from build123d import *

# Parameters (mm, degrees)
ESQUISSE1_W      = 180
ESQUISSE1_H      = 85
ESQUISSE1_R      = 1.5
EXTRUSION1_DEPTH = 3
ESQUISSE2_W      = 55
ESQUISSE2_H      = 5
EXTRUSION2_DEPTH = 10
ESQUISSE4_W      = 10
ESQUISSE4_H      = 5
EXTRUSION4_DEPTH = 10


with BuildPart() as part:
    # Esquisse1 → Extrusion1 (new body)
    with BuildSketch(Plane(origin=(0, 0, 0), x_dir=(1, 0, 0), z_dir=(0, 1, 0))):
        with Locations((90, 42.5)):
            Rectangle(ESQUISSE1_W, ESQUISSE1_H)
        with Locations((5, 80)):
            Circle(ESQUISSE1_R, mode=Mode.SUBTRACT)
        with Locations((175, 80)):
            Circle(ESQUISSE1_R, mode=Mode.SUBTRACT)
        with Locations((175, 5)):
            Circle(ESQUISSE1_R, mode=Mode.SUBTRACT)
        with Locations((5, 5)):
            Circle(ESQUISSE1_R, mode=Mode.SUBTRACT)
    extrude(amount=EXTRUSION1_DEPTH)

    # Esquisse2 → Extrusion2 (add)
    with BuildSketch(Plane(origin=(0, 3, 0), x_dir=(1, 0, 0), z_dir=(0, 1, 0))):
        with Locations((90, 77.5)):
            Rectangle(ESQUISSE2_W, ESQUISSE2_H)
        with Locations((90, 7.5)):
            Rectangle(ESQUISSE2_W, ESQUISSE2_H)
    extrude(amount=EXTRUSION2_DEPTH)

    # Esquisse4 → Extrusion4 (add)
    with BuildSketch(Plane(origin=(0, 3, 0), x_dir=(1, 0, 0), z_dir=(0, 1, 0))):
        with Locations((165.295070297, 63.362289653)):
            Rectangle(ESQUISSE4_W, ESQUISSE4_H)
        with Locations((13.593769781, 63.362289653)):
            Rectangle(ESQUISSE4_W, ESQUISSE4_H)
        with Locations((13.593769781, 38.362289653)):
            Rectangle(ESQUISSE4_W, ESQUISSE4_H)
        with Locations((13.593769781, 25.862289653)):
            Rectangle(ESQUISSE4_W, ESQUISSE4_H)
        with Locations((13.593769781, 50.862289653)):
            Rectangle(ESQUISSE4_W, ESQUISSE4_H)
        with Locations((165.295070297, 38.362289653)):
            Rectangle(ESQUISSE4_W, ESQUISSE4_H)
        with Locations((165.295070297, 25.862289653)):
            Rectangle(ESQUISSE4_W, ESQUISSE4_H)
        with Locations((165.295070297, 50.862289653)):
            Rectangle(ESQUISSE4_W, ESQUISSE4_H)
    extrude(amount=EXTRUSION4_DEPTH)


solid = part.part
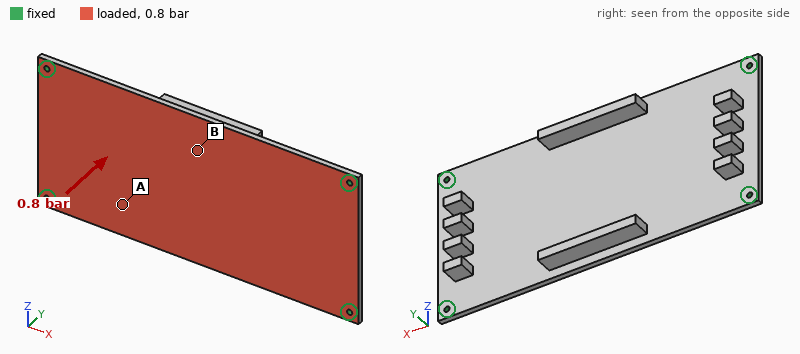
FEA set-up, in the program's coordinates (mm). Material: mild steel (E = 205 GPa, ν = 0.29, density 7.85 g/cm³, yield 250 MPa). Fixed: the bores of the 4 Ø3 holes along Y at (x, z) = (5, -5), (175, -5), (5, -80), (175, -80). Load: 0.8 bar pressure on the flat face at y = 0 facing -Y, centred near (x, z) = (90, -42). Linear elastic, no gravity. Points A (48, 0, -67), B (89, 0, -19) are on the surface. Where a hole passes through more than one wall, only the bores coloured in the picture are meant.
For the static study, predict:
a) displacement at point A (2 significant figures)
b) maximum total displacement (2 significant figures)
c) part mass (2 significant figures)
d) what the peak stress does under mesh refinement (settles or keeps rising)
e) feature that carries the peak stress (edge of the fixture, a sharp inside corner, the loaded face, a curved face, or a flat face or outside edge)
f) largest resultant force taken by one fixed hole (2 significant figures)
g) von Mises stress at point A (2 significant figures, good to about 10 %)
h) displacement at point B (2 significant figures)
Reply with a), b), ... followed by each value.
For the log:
a) 0.26 mm
b) 0.34 mm
c) 430 g
d) keeps rising
e) edge of the fixture
f) 330 N
g) 50 MPa
h) 0.33 mm
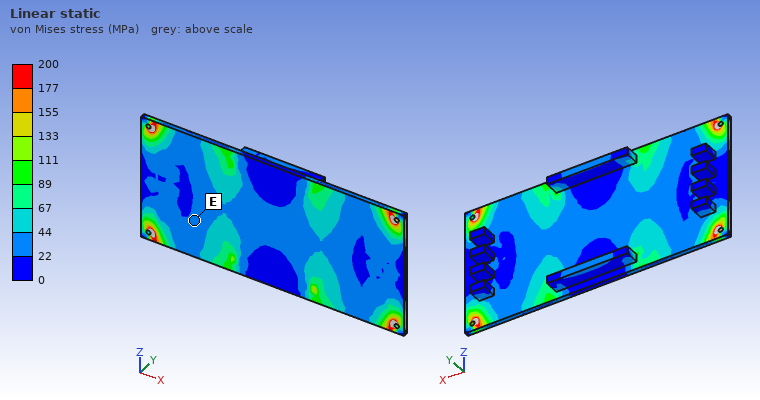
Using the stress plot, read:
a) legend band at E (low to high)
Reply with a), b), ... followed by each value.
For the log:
a) 22 to 44 MPa
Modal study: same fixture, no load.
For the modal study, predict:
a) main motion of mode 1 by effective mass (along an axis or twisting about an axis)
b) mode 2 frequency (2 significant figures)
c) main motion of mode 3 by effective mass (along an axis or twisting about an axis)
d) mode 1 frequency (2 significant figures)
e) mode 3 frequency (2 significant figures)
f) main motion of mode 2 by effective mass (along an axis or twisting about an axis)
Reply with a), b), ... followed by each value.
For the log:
a) along Y
b) 840 Hz
c) twisting about Z
d) 510 Hz
e) 1200 Hz
f) twisting about X
